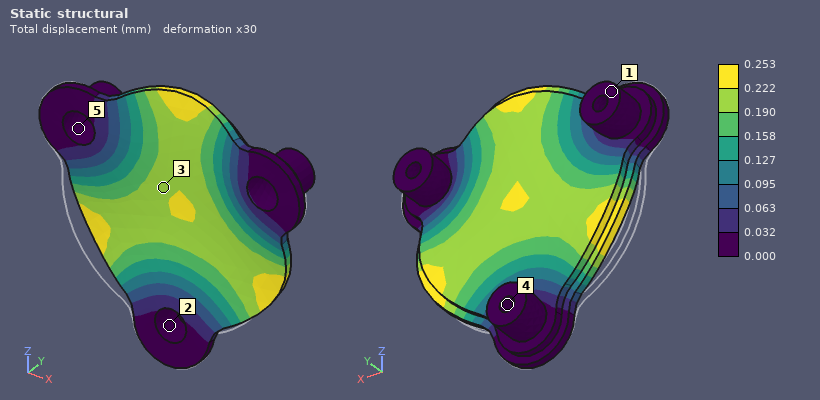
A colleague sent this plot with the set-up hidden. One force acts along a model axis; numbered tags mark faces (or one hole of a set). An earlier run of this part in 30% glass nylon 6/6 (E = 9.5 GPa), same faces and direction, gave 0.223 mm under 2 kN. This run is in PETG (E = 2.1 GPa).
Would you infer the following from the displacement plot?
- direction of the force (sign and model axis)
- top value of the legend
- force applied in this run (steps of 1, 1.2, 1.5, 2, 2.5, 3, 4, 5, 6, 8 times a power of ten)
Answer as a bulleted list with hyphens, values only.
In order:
- +Y
- 0.253 mm
- 500 N
